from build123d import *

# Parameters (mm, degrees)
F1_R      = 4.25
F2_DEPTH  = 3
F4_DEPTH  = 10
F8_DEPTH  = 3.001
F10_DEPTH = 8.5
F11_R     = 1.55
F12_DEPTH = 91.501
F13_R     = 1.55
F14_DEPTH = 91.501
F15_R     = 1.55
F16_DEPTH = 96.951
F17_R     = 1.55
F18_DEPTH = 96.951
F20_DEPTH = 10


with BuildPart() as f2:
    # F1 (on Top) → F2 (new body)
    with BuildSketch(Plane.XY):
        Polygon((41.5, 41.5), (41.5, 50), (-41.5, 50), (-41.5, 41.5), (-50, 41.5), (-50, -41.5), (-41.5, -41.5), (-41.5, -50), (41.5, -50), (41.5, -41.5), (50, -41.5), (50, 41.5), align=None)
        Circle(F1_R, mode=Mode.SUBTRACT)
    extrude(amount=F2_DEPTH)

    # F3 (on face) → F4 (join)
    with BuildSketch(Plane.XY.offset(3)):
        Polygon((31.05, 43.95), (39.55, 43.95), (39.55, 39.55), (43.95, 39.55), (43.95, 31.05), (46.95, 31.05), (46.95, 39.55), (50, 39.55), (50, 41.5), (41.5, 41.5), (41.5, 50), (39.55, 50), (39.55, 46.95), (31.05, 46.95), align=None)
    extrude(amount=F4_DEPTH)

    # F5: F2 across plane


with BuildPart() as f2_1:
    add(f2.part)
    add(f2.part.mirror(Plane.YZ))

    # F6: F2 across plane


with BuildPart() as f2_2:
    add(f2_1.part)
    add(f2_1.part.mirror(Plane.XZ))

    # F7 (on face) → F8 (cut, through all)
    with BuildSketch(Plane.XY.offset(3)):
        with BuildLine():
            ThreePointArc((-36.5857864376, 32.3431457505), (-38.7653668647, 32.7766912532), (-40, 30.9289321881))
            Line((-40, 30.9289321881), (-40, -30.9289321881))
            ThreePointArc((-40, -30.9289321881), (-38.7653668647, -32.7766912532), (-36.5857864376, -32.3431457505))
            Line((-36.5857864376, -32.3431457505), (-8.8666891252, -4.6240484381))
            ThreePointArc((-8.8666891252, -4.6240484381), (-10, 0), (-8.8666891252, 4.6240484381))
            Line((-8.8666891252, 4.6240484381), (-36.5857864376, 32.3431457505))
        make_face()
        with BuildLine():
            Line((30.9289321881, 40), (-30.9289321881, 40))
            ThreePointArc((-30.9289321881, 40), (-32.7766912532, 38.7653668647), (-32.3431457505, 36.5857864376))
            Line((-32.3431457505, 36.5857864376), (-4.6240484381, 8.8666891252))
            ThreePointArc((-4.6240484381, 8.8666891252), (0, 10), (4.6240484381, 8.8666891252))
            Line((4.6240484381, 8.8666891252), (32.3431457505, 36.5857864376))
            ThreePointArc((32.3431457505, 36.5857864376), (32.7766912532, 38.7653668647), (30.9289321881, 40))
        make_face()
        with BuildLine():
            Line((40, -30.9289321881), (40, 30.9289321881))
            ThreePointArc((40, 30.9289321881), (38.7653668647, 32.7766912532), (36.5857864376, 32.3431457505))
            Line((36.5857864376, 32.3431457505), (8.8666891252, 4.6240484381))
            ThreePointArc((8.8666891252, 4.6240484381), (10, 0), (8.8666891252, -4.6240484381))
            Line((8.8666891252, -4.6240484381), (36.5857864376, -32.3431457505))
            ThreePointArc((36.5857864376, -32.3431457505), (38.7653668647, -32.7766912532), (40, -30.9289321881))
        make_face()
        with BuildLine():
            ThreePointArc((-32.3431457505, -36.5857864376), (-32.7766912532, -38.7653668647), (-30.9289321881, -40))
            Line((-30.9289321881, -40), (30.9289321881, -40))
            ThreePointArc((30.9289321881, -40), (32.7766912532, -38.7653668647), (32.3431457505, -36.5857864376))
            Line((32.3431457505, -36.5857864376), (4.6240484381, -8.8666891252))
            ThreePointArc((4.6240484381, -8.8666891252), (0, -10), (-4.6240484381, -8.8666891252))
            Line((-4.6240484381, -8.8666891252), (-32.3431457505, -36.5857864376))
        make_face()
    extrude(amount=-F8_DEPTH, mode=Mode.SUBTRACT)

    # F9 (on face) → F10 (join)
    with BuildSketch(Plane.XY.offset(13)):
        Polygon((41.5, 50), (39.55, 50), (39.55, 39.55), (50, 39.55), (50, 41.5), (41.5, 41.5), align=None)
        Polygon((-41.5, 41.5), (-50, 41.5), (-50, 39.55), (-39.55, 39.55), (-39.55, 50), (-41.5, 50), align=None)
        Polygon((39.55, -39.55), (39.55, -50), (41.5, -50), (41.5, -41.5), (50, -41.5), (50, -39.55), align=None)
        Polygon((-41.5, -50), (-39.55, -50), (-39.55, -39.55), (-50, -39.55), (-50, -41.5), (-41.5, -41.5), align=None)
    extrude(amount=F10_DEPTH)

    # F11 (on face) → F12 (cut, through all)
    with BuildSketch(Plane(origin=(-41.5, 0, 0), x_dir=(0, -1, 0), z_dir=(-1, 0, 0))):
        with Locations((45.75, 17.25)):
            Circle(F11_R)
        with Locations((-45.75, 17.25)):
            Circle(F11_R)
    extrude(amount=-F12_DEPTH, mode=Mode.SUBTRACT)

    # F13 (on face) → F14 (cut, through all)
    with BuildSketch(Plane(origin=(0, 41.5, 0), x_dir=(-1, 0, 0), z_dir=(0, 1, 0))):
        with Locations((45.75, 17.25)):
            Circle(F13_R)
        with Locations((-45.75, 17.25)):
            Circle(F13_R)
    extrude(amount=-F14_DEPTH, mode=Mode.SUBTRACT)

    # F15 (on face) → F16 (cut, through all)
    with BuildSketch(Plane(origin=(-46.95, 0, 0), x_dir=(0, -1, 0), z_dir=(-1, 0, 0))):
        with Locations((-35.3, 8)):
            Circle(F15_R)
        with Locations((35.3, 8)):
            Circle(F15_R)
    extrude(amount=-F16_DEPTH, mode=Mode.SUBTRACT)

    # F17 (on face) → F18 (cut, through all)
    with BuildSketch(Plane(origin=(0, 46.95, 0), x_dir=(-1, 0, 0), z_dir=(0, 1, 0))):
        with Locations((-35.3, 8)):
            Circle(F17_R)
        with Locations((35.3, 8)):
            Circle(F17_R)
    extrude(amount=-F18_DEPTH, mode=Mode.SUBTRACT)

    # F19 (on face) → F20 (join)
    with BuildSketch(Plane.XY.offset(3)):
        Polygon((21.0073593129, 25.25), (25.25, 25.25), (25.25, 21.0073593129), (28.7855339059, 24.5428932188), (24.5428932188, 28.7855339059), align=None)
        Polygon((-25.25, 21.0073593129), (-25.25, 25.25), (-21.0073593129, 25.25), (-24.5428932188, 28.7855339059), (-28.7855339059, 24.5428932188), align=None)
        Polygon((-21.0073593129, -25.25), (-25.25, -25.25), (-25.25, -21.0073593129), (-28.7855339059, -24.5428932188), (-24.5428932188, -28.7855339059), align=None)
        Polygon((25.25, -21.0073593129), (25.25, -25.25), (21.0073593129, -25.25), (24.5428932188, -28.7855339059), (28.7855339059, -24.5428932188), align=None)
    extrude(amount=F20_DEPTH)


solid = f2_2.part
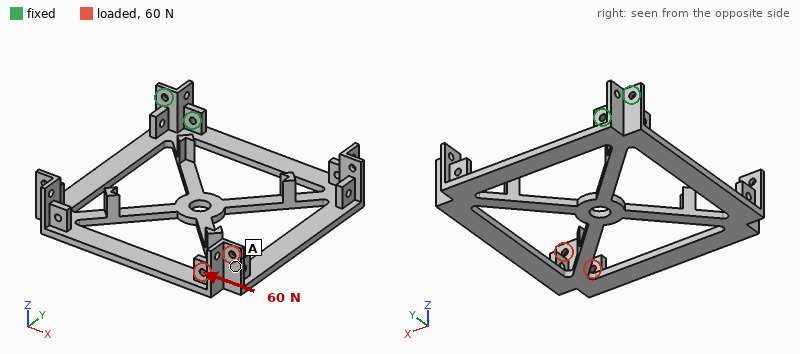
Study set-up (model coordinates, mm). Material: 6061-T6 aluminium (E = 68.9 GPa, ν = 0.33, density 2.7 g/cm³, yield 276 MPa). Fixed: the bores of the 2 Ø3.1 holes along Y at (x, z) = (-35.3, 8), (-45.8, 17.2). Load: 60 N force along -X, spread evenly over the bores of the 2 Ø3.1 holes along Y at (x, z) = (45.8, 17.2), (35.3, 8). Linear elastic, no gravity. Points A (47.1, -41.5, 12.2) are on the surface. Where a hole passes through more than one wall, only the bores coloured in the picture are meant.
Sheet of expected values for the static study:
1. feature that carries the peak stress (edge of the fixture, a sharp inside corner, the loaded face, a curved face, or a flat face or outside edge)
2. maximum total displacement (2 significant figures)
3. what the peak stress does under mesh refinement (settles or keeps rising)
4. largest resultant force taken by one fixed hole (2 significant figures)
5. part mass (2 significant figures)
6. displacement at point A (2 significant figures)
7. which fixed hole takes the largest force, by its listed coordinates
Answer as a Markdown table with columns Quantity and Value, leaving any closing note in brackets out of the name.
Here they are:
| Quantity | Value |
|---|---|
| feature that carries the peak stress | edge of the fixture |
| maximum total displacement | 1.3 mm |
| what the peak stress does under mesh refinement | keeps rising |
| largest resultant force taken by one fixed hole | 200 N |
| part mass | 52 g |
| displacement at point A | 1.2 mm |
| which fixed hole takes the largest force, by its listed coordinates | (-45.8, 17.2) |
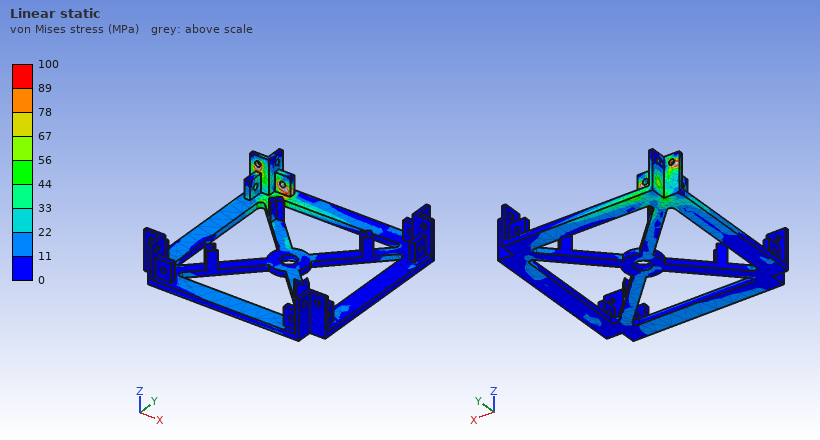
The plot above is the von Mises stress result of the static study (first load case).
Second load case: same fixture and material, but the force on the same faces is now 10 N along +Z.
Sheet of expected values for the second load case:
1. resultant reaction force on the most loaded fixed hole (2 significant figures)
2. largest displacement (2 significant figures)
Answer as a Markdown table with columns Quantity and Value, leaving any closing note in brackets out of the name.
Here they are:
| Quantity | Value |
|---|---|
| resultant reaction force on the most loaded fixed hole | 48 N |
| largest displacement | 1.6 mm |
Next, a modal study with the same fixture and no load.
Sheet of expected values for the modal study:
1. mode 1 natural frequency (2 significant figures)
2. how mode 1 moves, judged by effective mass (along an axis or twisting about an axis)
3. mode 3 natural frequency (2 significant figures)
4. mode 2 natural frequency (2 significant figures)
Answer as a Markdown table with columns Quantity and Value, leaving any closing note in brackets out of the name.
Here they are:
| Quantity | Value |
|---|---|
| mode 1 natural frequency | 110 Hz |
| how mode 1 moves, judged by effective mass | along Z |
| mode 3 natural frequency | 260 Hz |
| mode 2 natural frequency | 220 Hz |
